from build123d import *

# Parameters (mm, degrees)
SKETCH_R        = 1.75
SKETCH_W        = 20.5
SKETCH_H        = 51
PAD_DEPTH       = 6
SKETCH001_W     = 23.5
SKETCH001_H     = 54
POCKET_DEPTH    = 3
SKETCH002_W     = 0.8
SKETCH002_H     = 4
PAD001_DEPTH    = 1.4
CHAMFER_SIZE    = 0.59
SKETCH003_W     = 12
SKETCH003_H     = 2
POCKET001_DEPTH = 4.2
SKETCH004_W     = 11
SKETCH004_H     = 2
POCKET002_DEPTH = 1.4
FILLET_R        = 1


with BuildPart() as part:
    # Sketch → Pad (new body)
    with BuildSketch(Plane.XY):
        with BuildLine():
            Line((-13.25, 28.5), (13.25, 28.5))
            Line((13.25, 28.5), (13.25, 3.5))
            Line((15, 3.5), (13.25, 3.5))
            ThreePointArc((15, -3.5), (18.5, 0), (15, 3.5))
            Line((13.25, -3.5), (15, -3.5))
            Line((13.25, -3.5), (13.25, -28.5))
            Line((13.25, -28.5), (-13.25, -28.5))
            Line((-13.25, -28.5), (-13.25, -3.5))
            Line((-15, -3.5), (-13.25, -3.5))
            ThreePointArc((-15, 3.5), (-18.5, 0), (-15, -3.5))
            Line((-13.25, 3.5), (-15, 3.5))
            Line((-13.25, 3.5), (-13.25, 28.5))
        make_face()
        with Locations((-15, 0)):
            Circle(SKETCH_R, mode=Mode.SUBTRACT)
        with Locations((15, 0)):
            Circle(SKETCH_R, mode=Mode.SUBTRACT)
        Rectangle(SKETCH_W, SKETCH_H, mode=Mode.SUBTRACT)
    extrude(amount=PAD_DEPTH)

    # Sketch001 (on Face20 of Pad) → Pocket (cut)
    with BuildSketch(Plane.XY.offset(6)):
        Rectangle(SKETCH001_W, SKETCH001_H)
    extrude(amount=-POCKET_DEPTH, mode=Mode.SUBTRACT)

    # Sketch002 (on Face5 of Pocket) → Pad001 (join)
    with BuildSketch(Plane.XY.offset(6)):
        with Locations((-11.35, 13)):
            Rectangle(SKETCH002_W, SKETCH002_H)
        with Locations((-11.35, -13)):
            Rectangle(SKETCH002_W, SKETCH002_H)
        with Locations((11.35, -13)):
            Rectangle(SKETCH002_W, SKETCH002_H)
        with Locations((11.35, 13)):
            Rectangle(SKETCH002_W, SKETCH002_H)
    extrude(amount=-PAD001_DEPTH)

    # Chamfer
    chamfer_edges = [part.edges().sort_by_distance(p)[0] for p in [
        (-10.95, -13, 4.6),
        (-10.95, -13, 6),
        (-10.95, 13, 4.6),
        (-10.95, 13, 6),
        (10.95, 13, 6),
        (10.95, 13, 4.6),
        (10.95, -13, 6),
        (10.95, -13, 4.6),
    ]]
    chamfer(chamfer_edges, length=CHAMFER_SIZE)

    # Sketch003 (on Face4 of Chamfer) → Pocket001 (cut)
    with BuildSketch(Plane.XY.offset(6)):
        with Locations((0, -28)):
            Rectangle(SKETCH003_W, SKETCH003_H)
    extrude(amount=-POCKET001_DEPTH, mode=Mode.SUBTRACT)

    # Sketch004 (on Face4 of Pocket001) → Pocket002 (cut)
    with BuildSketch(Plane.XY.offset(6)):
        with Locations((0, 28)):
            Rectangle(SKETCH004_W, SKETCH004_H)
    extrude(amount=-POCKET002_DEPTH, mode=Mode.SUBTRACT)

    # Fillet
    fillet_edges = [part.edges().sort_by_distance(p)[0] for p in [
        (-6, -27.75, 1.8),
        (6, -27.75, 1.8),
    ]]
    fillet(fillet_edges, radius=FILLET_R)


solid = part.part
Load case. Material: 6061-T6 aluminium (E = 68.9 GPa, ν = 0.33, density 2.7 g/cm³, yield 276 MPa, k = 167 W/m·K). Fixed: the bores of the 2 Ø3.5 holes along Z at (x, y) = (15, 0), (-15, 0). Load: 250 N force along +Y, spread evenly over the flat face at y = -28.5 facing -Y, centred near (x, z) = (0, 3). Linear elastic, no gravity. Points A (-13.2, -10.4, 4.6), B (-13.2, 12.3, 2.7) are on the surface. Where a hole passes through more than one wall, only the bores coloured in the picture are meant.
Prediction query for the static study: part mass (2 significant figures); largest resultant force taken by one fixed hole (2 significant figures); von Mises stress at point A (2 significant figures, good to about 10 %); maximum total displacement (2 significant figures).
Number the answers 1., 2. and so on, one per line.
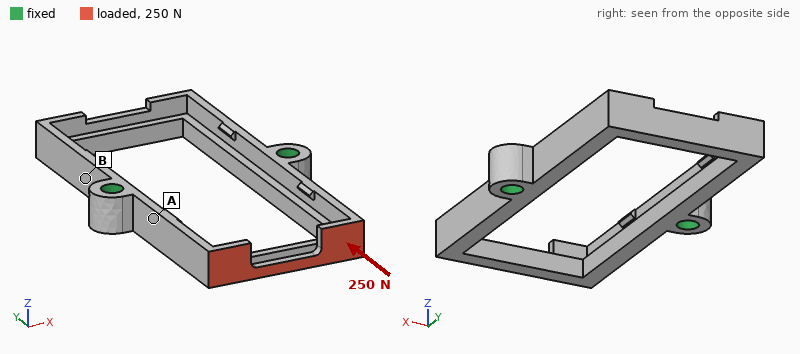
1. 6.2 g
2. 130 N
3. 9.4 MPa
4. 35 µm
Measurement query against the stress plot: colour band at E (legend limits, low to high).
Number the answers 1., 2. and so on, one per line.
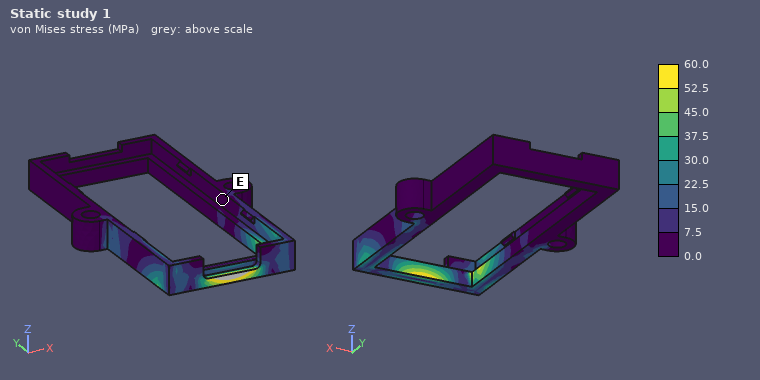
1. 0.0 to 7.5 MPa
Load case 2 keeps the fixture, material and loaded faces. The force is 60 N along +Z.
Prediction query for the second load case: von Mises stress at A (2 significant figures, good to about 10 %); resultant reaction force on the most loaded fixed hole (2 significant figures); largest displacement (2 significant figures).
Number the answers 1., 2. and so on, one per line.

1. 27 MPa
2. 30 N
3. 99 µm
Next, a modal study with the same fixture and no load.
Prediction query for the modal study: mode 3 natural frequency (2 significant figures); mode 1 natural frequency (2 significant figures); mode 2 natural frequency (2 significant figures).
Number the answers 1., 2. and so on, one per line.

1. 3900 Hz
2. 3300 Hz
3. 3400 Hz
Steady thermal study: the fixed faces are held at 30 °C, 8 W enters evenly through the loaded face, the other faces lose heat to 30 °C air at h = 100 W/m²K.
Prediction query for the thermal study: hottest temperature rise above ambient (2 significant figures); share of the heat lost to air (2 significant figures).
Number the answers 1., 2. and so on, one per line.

1. 39 K
2. 31 %
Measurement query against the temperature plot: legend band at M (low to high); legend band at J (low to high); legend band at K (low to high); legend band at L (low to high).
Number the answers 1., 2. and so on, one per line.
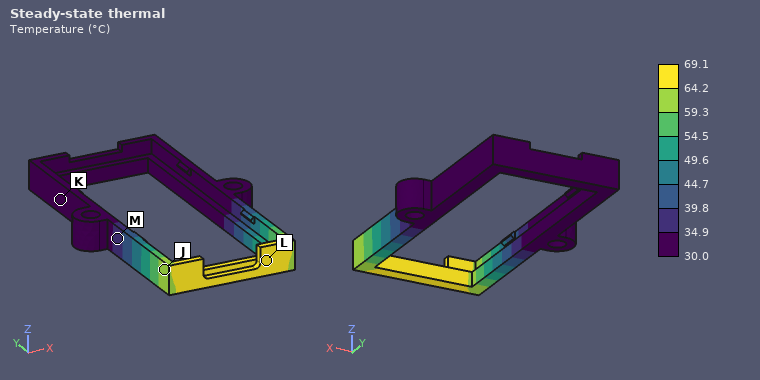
1. 34.9 to 39.8 °C
2. 59.3 to 64.2 °C
3. 30.0 to 34.9 °C
4. 64.2 to 69.1 °C
